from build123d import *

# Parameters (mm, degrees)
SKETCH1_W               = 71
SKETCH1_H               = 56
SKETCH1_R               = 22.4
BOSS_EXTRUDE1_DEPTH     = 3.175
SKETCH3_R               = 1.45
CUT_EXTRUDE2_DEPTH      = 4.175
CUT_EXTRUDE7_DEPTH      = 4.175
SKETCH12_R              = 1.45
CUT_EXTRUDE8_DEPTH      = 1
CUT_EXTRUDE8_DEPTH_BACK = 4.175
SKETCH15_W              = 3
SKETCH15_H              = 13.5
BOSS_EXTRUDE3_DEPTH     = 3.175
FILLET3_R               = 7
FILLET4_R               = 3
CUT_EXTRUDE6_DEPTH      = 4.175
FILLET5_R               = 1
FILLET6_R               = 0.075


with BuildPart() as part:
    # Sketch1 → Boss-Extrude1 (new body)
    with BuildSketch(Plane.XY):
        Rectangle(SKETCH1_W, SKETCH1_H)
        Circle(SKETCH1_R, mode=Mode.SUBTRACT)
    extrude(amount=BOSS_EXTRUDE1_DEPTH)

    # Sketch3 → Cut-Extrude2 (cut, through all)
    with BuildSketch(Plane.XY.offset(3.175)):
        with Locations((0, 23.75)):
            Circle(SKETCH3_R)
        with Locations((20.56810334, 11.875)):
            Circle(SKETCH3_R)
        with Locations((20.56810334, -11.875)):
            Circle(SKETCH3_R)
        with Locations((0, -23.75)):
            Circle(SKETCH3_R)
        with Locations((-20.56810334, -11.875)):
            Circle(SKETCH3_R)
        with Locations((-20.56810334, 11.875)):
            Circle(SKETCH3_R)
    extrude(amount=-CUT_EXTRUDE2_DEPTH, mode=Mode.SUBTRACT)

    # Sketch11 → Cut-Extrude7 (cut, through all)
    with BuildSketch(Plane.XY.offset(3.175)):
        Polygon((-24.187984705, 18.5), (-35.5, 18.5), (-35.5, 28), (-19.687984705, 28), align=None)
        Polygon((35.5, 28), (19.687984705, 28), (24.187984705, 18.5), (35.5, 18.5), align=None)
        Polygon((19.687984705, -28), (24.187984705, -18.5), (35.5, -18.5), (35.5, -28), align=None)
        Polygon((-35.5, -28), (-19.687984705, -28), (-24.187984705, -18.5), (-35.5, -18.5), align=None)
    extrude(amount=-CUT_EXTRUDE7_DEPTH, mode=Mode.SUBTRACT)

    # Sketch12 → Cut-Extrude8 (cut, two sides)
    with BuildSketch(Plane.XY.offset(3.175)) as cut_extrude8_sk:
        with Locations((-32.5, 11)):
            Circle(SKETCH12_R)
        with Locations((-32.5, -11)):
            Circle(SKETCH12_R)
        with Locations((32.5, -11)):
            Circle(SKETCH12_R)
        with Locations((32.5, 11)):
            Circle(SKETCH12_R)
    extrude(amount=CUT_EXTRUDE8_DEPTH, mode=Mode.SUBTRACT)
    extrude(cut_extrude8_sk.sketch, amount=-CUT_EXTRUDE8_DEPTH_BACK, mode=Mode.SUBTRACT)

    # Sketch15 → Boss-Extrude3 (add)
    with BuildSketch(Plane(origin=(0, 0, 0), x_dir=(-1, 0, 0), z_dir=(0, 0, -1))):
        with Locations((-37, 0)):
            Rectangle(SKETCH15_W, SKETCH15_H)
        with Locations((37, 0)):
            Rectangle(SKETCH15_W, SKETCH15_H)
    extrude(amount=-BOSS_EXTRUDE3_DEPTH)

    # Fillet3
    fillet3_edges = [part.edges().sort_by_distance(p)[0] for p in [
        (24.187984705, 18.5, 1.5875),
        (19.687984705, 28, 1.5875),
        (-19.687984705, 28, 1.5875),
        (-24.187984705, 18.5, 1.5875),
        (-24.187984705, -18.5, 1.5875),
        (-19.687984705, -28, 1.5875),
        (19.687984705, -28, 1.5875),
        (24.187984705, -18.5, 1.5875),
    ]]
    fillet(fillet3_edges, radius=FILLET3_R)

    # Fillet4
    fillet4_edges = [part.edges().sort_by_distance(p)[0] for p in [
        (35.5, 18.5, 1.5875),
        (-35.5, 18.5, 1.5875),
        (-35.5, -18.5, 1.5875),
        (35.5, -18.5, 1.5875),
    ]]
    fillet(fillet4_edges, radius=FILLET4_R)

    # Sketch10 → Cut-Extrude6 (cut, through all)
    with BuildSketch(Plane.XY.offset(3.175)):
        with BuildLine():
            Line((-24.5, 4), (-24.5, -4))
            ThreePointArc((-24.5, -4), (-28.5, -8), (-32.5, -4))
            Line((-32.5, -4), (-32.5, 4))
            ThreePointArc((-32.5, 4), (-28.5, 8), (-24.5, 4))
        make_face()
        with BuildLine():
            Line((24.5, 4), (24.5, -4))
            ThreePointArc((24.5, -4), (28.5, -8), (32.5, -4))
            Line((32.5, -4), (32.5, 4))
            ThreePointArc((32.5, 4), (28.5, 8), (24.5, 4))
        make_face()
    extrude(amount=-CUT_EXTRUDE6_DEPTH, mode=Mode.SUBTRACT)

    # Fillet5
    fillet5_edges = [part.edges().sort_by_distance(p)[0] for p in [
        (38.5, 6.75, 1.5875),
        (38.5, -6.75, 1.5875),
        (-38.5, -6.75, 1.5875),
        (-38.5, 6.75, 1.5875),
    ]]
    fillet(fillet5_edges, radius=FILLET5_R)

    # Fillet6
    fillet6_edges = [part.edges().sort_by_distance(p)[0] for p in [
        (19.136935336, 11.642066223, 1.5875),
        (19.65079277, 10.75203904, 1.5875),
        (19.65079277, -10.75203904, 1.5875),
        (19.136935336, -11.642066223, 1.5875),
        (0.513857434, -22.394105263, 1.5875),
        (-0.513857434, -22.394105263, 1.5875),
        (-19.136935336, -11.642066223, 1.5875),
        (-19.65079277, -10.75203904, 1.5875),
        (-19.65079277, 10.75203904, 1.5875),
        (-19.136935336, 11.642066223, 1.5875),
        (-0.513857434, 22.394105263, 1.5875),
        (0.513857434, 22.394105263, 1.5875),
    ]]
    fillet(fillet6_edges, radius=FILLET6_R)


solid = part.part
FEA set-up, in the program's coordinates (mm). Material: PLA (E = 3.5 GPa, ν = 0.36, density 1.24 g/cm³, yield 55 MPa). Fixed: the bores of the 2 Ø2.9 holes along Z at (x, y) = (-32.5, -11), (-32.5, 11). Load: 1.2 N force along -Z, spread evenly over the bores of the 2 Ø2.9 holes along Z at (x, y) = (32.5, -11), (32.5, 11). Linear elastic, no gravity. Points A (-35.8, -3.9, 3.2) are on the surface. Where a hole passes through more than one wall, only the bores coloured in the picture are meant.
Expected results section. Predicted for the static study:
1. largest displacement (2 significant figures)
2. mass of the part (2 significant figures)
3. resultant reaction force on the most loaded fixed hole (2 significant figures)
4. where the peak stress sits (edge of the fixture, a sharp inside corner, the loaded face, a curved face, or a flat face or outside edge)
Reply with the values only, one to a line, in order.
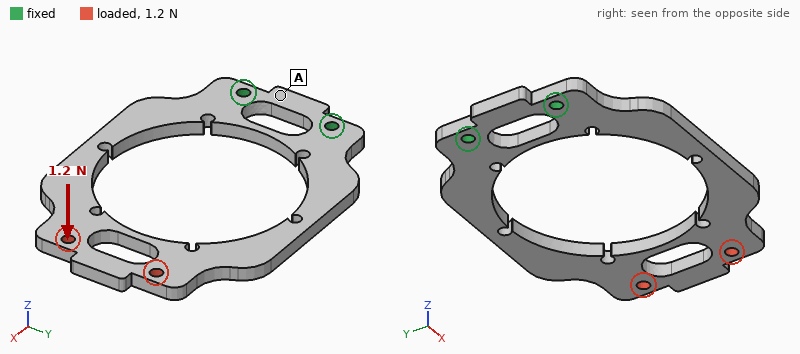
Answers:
0.97 mm
6.5 g
0.60 N
a curved face
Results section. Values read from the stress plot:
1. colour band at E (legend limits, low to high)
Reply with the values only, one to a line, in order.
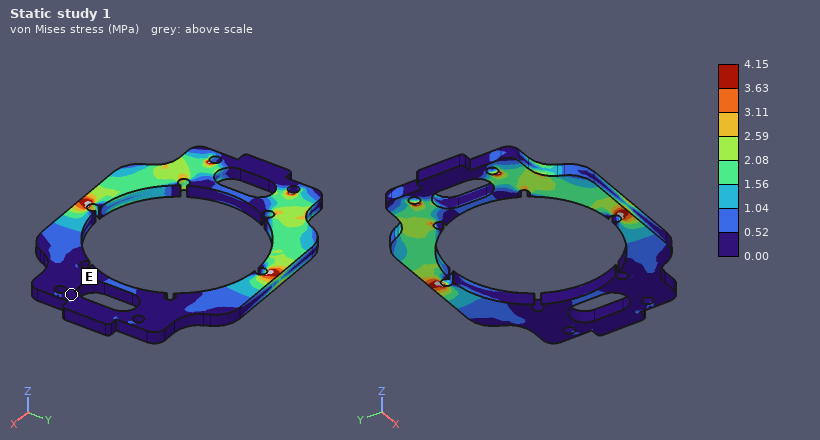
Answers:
0.00 to 0.52 MPa
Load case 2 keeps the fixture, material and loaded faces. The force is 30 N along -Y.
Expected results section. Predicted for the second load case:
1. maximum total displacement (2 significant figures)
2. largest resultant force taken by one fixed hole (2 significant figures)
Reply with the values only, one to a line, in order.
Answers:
1.1 mm
42 N
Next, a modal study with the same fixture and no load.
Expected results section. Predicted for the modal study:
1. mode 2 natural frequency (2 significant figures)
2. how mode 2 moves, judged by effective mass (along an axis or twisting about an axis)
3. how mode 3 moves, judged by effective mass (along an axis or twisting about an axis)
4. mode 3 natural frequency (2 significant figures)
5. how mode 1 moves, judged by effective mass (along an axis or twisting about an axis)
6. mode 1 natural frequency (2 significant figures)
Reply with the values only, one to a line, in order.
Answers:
380 Hz
twisting about X
along Y
510 Hz
along Z
130 Hz
